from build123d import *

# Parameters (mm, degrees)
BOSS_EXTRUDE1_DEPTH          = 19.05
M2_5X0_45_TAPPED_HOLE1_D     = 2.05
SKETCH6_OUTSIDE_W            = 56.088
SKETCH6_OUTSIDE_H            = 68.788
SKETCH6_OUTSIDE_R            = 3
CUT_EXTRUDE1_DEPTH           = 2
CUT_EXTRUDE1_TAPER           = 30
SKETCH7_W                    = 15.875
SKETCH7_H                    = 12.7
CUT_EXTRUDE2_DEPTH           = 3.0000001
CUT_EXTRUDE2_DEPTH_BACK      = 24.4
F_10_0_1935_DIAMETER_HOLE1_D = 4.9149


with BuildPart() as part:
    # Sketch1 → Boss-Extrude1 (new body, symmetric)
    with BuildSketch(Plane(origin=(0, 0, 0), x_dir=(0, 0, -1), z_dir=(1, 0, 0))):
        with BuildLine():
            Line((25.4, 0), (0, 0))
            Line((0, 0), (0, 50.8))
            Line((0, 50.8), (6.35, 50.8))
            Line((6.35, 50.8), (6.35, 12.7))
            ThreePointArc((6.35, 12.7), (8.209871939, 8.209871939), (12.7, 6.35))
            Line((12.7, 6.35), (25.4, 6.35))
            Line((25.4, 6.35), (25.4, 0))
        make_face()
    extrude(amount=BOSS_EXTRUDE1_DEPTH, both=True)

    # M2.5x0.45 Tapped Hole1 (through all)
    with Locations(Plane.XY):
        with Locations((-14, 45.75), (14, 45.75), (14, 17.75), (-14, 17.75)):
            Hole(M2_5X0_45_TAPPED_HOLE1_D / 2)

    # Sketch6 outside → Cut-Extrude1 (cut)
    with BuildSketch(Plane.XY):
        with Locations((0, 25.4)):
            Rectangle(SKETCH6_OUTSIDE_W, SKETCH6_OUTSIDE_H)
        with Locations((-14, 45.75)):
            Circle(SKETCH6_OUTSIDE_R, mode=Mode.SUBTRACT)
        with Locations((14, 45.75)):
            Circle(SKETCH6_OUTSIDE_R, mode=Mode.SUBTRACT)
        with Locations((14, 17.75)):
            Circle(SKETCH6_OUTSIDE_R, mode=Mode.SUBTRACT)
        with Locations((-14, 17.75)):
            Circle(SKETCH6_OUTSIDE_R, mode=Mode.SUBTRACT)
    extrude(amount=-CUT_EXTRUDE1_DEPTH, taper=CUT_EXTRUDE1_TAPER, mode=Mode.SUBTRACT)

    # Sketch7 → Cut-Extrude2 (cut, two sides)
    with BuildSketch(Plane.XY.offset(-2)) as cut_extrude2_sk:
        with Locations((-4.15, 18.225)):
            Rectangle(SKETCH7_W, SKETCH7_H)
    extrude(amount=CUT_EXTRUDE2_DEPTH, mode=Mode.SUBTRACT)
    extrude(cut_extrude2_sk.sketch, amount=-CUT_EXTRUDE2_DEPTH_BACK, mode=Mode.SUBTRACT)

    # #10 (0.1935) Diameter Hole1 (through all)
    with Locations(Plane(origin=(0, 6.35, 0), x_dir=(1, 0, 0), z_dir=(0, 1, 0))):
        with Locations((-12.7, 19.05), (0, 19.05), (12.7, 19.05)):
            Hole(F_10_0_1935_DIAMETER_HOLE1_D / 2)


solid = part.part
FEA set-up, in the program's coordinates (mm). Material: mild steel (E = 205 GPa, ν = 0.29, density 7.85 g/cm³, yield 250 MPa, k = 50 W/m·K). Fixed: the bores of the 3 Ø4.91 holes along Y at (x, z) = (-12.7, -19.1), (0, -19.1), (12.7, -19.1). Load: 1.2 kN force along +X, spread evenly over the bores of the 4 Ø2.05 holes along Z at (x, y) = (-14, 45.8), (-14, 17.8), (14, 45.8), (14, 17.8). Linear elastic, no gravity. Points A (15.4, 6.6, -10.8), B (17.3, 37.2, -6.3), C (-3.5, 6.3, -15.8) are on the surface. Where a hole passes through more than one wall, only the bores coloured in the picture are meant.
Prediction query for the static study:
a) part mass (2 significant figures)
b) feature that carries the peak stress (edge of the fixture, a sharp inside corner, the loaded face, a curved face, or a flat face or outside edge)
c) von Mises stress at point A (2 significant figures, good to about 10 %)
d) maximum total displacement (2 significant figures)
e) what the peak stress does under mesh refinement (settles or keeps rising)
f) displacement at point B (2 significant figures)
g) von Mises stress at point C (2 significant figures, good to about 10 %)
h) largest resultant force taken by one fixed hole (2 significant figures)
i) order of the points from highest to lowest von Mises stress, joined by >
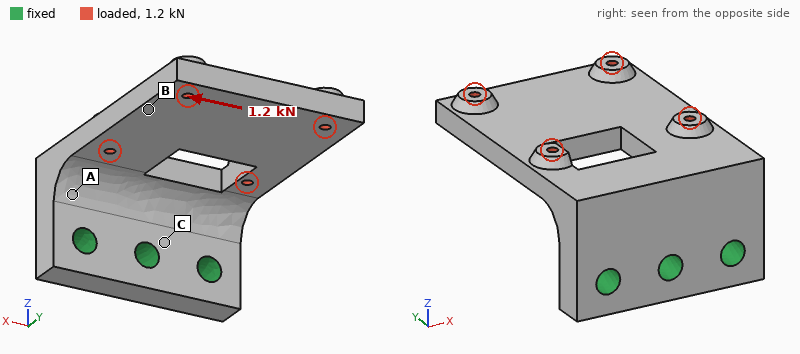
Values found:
97 g
edge of the fixture
54 MPa
45 µm
keeps rising
35 µm
39 MPa
1.4 kN
A > C > B
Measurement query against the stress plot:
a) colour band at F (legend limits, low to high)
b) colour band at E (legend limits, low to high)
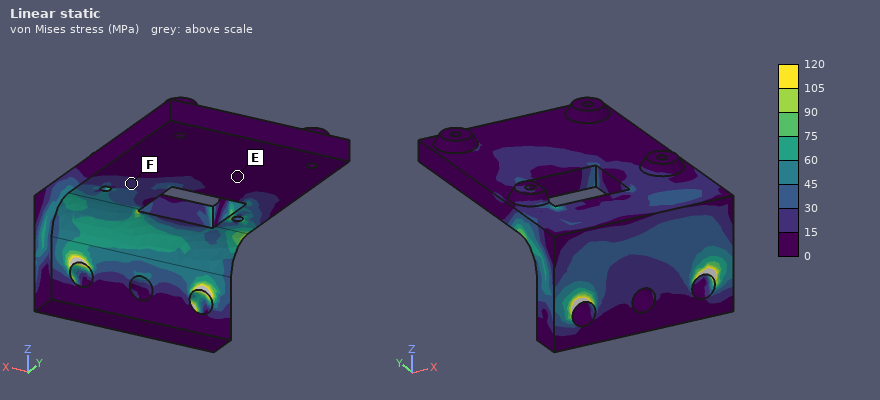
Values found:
15 to 30 MPa
0 to 15 MPa
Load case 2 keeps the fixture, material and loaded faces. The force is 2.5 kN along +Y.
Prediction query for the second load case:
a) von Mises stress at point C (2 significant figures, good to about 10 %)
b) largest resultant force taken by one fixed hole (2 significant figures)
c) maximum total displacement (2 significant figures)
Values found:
90 MPa
880 N
0.12 mm
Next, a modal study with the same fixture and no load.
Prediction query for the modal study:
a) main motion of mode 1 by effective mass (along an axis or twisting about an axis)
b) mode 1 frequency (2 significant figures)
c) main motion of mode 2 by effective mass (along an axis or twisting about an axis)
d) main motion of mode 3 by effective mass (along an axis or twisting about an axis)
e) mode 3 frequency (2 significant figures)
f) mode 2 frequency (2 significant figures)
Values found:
along Z
1400 Hz
along X
along X
4800 Hz
3800 Hz
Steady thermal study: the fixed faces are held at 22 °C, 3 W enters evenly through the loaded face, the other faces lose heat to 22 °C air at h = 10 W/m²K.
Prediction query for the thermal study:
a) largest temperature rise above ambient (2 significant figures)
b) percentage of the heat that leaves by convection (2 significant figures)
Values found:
15 K
14 %
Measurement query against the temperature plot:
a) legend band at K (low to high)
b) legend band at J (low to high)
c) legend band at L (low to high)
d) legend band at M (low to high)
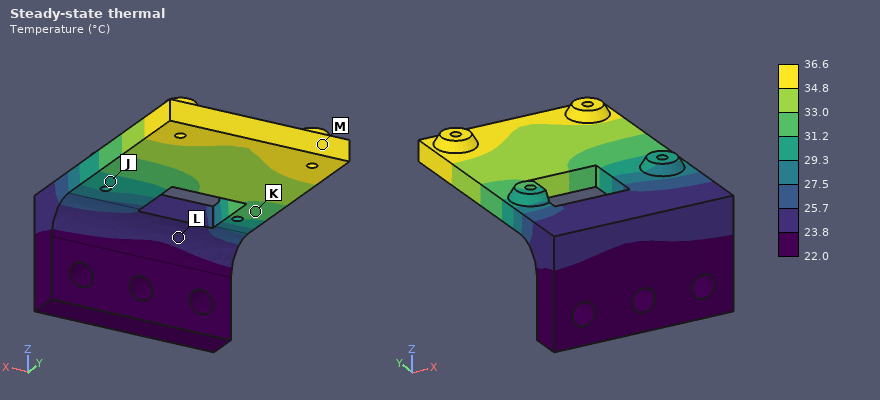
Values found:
31.2 to 33.0 °C
29.3 to 31.2 °C
23.8 to 25.7 °C
34.8 to 36.6 °C
